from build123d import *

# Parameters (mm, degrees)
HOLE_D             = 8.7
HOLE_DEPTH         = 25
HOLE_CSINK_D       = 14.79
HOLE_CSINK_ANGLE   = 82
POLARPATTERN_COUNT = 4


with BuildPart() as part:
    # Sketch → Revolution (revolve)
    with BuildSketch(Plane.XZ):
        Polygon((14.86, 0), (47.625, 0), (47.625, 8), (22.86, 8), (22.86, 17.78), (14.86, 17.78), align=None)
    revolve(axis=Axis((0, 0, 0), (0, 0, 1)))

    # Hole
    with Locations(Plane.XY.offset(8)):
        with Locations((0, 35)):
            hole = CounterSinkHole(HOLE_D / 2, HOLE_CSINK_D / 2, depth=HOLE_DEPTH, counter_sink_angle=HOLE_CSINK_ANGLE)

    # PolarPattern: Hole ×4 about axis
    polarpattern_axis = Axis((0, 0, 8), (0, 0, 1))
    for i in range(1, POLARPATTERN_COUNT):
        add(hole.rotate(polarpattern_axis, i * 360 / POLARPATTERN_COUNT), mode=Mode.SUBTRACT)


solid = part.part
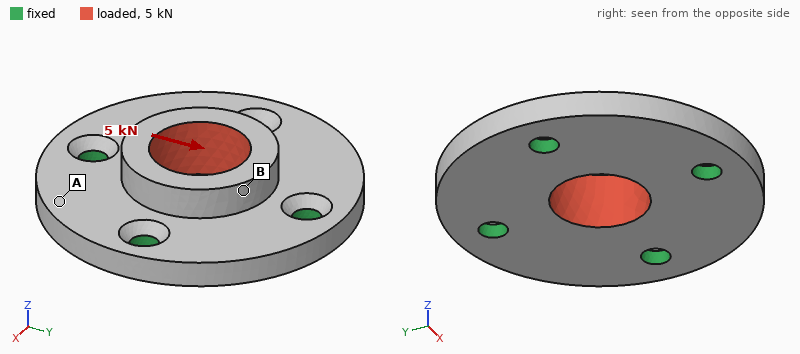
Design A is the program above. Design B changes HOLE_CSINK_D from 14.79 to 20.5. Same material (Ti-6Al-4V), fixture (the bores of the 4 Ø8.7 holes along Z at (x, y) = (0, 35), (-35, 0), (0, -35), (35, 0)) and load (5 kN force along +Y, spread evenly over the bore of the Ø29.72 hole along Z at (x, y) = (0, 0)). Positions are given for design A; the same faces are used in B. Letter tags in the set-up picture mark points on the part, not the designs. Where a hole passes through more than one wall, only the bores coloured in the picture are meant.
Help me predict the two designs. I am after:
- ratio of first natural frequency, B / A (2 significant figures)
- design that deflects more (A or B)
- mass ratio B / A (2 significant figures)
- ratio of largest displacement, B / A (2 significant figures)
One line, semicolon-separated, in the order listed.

0.80; B; 0.96; 1.6
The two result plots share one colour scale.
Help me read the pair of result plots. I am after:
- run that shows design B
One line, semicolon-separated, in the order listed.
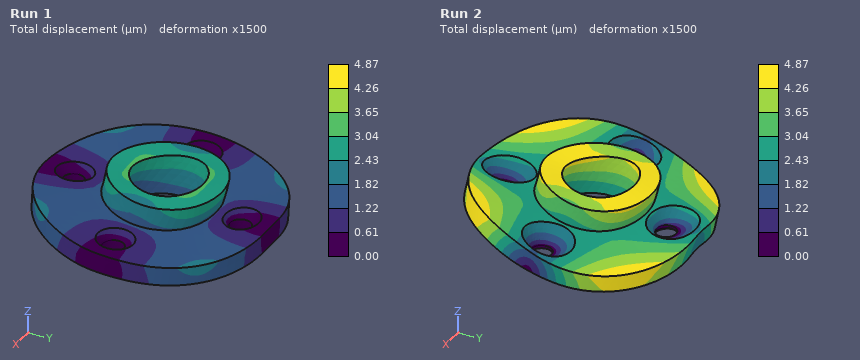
Run 2
